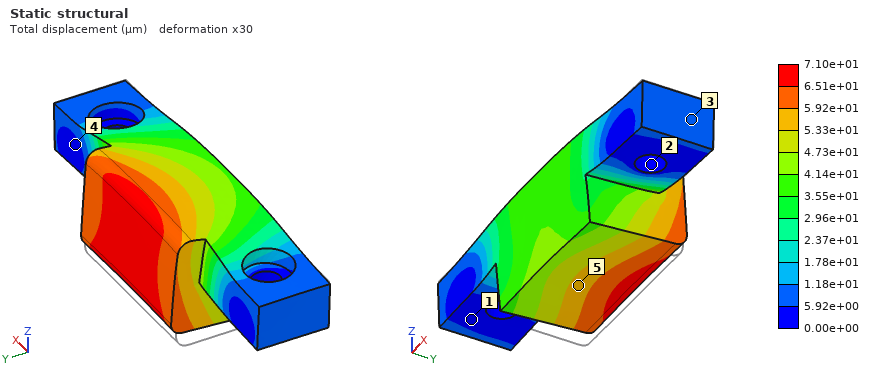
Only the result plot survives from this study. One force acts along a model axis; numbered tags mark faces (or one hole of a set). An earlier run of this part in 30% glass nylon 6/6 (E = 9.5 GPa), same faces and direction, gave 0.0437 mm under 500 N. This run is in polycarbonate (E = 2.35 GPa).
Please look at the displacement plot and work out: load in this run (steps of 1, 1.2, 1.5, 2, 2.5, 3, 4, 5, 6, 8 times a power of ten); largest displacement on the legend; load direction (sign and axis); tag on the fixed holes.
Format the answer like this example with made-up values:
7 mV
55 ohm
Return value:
200 N
7.10e+01 µm
+Z
2
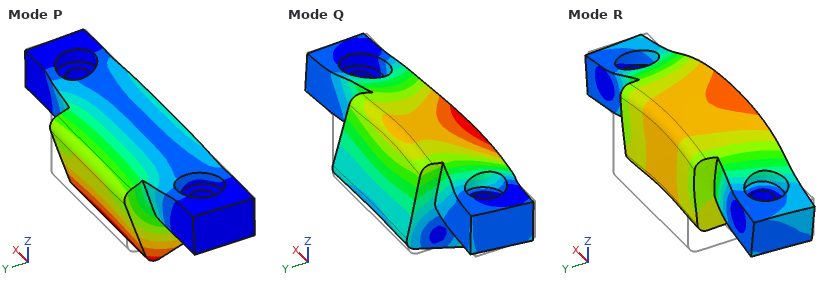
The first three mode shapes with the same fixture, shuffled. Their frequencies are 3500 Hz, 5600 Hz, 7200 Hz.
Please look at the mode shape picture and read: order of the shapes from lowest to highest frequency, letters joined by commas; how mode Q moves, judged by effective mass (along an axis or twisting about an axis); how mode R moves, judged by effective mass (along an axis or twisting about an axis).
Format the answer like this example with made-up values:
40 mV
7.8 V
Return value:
P, R, Q
along Y
along Z
